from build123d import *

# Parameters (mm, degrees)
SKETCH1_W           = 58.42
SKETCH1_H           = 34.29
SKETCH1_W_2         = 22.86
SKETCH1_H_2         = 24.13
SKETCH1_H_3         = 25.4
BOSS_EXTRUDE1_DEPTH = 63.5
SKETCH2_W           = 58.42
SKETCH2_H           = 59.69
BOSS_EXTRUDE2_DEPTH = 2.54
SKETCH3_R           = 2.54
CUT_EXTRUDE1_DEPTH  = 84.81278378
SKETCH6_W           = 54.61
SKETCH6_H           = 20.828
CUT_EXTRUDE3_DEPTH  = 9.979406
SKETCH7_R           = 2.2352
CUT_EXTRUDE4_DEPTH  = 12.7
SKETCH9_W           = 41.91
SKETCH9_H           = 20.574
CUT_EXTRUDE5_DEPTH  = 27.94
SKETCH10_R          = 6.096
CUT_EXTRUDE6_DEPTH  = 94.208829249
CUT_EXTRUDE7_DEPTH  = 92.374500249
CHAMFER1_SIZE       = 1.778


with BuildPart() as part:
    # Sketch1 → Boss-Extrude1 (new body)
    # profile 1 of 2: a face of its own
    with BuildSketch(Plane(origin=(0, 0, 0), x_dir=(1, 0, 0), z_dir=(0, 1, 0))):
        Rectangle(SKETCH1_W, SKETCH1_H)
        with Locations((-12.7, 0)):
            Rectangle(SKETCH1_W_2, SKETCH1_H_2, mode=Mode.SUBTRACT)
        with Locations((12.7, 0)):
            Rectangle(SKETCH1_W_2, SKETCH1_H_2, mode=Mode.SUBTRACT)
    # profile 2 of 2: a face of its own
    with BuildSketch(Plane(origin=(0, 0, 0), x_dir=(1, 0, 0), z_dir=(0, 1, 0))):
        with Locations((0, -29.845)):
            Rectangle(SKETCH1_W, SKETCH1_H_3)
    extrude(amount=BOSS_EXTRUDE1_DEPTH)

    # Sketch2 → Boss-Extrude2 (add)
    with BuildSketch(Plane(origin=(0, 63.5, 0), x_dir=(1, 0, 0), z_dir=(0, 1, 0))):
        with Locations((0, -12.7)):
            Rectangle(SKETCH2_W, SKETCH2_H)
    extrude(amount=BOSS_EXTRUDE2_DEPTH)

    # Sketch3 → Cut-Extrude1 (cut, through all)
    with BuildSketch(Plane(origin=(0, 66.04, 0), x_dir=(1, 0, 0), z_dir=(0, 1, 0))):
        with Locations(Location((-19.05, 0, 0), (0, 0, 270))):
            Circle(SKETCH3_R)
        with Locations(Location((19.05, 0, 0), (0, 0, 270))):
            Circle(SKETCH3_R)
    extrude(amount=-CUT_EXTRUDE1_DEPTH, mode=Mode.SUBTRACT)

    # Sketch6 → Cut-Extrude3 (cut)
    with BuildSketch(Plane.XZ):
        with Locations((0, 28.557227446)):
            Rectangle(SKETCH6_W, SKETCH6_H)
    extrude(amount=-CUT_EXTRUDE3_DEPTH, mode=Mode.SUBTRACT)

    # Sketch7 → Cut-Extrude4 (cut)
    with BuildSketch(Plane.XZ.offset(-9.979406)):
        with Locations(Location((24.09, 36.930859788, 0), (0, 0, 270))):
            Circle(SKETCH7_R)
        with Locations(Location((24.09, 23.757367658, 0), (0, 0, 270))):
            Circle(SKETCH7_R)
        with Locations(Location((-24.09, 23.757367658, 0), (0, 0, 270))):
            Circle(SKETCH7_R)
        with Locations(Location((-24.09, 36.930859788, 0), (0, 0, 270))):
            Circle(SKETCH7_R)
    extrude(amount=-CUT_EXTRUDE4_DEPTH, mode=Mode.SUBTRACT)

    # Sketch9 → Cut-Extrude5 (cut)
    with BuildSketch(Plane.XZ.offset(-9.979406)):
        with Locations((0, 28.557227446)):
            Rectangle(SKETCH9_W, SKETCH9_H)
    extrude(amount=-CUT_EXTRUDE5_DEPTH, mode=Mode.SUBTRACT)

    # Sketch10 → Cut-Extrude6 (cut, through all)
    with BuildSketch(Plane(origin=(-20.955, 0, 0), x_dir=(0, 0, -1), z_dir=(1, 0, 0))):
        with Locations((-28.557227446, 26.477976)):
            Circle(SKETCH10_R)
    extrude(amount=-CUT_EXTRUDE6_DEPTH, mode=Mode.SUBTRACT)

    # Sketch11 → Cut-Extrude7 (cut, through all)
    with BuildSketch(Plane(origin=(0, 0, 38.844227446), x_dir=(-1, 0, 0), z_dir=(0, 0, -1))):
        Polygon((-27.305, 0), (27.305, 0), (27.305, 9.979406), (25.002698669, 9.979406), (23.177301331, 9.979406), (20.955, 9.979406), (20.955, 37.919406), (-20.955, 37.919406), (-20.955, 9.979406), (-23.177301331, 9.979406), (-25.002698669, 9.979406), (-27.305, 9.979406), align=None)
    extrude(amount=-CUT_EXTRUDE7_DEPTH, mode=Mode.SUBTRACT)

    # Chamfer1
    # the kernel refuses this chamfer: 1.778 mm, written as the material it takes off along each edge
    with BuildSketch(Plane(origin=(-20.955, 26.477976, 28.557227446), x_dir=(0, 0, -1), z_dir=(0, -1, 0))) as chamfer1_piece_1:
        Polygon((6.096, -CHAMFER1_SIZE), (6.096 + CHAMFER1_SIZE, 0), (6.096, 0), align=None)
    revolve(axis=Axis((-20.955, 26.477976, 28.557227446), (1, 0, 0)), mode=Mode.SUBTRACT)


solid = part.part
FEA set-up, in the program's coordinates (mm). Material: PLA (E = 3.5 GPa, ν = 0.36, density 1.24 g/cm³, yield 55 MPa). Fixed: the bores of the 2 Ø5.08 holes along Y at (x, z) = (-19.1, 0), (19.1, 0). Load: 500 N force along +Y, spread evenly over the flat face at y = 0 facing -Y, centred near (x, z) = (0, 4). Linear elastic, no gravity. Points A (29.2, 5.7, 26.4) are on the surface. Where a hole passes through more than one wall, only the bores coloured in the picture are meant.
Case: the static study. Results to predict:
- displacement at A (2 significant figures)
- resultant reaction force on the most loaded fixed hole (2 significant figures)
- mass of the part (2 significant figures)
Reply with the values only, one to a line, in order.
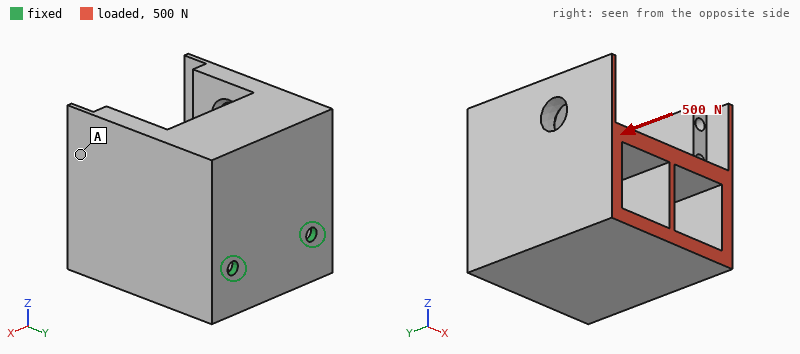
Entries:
0.77 mm
250 N
140 g
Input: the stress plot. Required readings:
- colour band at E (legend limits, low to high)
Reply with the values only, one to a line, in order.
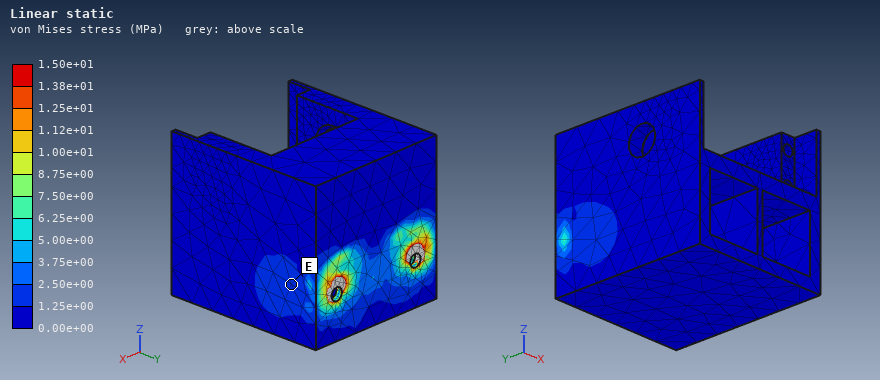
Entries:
1.25e+00 to 2.50e+00 MPa
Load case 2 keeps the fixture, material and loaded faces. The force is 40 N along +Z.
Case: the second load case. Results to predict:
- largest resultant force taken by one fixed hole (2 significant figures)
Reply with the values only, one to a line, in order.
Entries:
20 N
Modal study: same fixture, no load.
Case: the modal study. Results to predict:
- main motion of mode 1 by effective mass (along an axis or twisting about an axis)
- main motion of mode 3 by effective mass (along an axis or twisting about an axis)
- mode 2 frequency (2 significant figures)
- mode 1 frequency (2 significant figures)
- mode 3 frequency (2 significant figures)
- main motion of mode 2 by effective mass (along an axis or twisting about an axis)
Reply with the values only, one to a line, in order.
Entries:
along Z
along Y
610 Hz
140 Hz
1200 Hz
along X
